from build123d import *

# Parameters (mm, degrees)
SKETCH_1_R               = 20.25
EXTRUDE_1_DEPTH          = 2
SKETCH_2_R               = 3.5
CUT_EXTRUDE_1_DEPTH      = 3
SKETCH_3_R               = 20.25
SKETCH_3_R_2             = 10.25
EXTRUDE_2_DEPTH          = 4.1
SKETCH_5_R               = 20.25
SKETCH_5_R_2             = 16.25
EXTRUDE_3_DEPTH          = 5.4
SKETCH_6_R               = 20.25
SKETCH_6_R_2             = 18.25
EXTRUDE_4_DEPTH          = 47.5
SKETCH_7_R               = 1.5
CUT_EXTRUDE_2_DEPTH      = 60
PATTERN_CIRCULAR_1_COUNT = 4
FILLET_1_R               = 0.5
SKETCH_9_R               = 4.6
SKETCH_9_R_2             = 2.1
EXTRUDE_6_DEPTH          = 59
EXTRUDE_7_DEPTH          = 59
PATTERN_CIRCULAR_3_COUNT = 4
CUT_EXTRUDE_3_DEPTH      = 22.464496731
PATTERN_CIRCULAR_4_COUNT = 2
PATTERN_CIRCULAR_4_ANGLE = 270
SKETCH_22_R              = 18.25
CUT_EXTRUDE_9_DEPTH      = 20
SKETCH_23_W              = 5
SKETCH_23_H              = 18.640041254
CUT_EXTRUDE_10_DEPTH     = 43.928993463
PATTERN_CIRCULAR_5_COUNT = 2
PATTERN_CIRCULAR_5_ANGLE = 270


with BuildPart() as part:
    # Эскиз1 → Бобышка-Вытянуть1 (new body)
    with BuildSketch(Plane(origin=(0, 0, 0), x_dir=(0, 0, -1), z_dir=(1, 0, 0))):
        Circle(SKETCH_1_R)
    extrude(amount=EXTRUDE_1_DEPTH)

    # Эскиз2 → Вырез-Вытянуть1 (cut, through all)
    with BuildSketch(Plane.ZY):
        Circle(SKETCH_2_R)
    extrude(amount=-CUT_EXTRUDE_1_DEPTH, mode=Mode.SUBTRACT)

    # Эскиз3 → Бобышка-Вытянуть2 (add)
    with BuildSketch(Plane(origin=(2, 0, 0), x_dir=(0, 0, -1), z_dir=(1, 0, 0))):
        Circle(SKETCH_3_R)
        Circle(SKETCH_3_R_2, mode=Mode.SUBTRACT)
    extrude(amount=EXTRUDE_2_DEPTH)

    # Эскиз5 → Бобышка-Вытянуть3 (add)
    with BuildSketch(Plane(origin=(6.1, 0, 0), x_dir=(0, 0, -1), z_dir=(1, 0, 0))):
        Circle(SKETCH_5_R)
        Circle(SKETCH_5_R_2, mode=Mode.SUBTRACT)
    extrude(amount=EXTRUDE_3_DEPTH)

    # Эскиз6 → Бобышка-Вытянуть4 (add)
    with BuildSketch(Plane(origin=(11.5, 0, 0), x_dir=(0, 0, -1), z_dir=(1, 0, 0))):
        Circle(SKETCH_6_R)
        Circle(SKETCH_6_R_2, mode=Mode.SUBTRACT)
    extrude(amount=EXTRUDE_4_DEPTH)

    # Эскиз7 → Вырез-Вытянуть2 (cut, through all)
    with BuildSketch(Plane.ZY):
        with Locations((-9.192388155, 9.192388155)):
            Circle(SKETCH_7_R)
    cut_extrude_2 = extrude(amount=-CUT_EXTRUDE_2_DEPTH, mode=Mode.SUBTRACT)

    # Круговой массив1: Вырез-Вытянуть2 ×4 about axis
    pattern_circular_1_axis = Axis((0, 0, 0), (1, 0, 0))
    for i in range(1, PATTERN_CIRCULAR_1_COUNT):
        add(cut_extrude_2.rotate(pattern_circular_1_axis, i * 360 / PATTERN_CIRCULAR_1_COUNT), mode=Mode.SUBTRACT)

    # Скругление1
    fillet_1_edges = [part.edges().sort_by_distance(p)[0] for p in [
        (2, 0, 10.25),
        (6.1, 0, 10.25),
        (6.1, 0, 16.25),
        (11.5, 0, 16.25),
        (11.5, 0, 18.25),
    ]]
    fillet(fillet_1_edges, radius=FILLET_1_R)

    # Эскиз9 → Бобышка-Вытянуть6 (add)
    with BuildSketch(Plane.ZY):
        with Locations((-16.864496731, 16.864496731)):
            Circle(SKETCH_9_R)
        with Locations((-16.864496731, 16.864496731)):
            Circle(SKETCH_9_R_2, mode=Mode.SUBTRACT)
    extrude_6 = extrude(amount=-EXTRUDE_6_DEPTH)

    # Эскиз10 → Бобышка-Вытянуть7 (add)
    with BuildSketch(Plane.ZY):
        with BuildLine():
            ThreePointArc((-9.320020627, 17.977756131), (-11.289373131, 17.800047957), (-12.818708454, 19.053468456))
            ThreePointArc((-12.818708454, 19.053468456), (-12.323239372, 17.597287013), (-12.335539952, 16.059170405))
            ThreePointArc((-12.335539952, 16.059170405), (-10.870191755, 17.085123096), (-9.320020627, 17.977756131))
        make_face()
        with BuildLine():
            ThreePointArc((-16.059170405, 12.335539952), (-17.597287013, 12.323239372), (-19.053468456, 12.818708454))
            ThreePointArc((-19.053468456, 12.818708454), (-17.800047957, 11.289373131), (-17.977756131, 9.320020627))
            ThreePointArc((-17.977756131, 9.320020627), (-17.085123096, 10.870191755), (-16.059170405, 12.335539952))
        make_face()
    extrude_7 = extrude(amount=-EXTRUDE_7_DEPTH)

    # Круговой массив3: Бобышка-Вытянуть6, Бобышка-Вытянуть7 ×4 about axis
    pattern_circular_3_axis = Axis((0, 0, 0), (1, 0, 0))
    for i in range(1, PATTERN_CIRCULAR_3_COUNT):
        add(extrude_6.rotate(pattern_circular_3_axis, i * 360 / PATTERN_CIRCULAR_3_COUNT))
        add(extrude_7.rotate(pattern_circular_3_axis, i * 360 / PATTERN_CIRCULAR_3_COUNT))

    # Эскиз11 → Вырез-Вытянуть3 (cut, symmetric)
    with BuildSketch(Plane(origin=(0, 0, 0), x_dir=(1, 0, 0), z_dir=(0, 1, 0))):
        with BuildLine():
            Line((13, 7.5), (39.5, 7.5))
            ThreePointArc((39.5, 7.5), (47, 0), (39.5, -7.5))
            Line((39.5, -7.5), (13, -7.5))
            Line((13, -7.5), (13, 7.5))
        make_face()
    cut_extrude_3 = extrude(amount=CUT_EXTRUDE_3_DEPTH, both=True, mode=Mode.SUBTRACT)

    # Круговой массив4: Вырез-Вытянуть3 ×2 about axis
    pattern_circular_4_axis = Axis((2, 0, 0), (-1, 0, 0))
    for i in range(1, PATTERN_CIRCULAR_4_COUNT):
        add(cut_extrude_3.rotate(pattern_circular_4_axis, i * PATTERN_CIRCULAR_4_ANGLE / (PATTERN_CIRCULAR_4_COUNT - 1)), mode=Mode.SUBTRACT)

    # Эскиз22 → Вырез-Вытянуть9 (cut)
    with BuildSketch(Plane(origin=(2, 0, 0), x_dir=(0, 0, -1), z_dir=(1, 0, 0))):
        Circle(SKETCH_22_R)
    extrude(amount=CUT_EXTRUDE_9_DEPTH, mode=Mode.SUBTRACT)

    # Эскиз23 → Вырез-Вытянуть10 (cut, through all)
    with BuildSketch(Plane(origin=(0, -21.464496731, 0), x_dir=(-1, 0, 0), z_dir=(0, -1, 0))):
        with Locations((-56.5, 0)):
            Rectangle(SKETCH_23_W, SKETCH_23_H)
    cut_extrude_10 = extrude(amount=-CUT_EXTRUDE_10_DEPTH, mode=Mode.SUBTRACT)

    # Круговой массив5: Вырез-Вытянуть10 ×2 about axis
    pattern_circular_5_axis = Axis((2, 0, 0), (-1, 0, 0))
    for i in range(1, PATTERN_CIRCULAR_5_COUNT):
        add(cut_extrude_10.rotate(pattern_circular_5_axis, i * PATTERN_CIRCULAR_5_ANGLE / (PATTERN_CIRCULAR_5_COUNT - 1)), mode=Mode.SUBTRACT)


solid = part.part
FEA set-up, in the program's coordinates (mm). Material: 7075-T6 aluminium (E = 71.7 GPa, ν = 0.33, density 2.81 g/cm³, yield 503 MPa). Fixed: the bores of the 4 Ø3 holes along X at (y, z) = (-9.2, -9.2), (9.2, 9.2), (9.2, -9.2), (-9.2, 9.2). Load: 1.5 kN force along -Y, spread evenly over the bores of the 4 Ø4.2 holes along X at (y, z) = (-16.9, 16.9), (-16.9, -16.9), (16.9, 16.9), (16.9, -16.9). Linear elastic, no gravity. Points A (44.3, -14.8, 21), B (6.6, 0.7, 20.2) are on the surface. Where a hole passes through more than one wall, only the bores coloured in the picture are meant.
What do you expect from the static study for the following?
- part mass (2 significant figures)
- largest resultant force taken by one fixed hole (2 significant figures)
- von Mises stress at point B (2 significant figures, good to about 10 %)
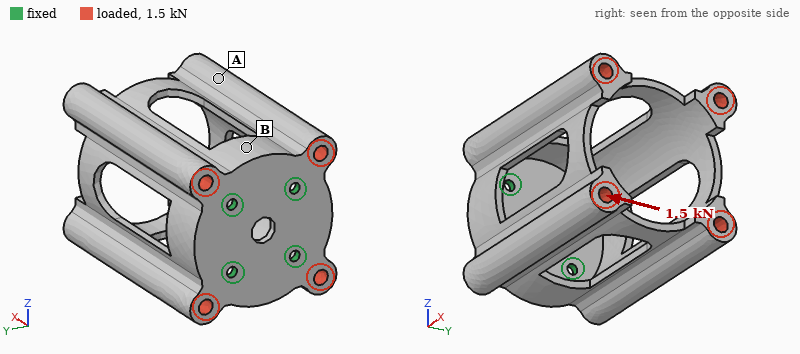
68 g
1.0 kN
48 MPa
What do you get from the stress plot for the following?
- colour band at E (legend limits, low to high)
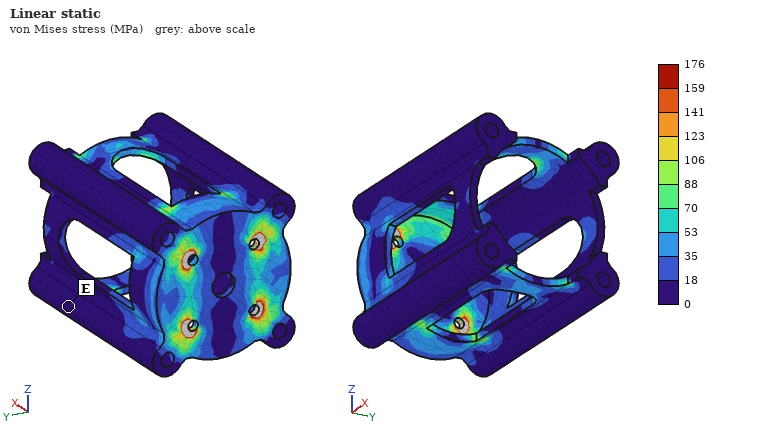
0 to 18 MPa
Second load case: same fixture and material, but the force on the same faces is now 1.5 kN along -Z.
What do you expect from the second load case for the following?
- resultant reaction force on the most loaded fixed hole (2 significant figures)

1.0 kN
